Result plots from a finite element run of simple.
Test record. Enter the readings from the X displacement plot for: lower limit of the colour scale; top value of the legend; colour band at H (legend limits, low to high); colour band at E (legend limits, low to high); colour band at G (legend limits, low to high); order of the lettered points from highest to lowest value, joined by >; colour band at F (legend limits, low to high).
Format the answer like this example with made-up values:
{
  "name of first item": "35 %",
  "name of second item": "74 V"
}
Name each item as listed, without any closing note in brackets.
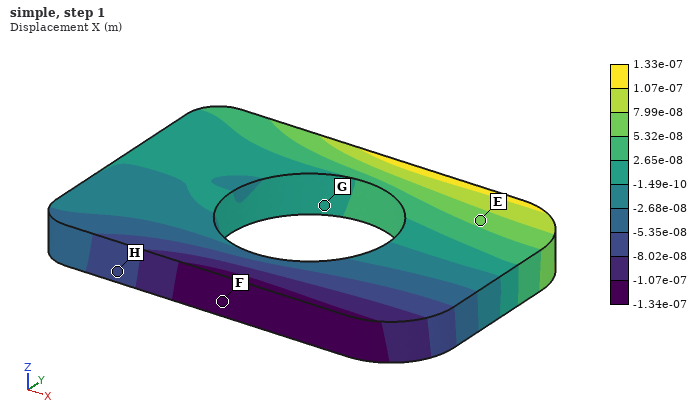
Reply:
{
  "lower limit of the colour scale": "-1.34e-07 m",
  "top value of the legend": "1.33e-07 m",
  "colour band at H": "-8.02e-08 to -5.35e-08 m",
  "colour band at E": "5.32e-08 to 7.99e-08 m",
  "colour band at G": "-1.49e-10 to 2.65e-08 m",
  "order of the lettered points from highest to lowest value, joined by >": "E > G > H > F",
  "colour band at F": "-1.34e-07 to -1.07e-07 m"
}
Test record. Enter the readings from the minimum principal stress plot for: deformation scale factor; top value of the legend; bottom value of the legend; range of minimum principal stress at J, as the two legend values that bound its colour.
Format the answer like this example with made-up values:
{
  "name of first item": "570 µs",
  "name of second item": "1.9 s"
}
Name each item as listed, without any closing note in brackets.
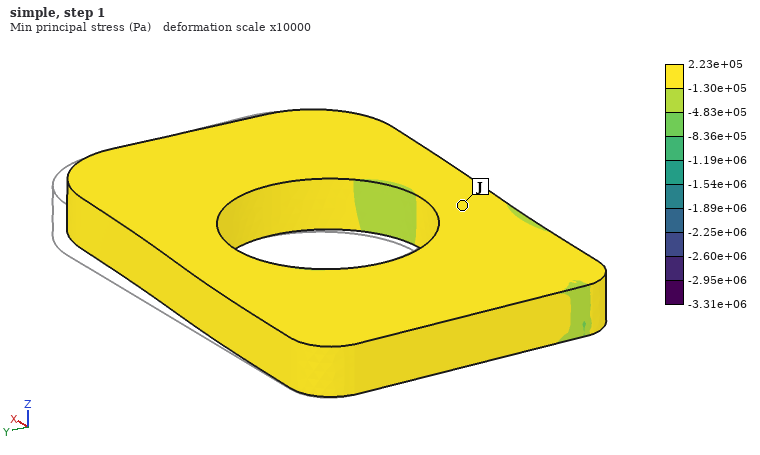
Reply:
{
  "deformation scale factor": "10000",
  "top value of the legend": "2.23e+05 Pa",
  "bottom value of the legend": "-3.31e+06 Pa",
  "range of minimum principal stress at J, as the two legend values that bound its colour": "-1.30e+05 to 2.23e+05 Pa"
}
